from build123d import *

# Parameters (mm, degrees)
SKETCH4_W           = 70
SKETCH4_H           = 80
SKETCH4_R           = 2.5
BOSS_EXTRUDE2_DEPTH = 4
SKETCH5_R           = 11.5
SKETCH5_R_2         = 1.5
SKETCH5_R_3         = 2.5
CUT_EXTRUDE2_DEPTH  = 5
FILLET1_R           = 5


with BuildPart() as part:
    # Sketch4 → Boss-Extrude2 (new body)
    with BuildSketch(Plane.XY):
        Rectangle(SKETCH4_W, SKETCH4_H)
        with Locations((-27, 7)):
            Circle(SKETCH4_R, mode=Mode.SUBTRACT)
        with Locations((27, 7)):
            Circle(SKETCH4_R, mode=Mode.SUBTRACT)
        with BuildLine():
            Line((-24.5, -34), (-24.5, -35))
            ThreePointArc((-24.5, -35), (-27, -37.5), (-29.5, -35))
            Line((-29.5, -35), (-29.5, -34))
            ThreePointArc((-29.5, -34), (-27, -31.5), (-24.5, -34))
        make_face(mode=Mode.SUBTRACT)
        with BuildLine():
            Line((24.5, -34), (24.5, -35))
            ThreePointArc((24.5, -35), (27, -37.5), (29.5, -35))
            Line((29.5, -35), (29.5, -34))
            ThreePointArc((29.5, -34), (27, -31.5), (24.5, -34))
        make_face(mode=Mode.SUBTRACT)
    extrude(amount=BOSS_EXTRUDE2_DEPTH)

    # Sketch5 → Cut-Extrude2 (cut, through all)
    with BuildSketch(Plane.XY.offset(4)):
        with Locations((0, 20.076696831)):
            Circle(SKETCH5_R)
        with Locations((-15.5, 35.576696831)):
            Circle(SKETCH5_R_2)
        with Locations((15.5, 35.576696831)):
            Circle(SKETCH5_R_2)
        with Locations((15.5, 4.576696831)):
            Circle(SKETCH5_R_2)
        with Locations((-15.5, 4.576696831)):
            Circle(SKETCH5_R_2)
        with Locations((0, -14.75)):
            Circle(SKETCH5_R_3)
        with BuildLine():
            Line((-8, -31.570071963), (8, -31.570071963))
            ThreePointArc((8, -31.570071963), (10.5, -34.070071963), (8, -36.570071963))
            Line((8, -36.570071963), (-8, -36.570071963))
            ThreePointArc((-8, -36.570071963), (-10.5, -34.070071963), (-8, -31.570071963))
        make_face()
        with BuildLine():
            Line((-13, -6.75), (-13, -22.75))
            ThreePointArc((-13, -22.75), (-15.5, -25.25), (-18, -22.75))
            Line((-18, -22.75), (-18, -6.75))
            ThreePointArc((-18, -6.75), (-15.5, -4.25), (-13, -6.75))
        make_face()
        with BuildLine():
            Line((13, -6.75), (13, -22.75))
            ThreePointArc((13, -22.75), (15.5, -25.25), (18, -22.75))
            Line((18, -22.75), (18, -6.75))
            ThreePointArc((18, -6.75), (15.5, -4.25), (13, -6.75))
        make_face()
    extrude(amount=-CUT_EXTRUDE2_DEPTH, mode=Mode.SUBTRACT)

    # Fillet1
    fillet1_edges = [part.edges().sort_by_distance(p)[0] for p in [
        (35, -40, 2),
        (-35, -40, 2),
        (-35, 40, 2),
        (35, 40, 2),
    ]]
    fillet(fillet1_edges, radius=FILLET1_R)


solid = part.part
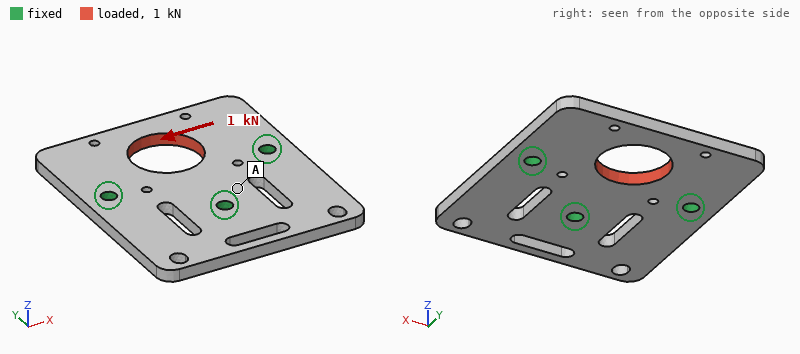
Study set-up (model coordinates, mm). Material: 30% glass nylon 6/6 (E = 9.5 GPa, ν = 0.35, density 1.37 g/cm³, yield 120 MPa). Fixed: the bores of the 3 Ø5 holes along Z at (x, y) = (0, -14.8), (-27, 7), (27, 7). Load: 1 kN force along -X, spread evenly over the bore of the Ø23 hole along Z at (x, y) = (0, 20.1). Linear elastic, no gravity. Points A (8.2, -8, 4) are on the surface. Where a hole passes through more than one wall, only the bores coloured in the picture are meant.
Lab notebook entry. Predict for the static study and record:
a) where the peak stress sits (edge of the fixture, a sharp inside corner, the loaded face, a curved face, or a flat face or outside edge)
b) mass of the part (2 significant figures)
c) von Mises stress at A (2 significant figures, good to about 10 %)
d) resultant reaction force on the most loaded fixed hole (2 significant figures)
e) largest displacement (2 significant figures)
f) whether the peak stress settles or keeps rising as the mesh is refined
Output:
edge of the fixture
26 g
1.9 MPa
510 N
52 µm
keeps rising
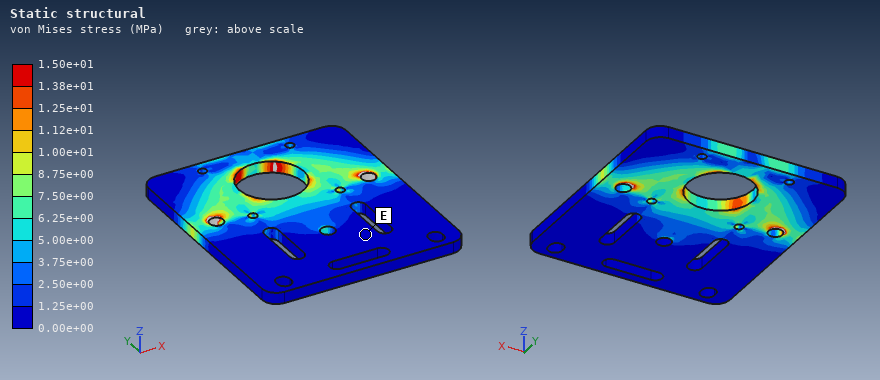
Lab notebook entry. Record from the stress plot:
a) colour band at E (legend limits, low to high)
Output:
0.00e+00 to 1.25e+00 MPa
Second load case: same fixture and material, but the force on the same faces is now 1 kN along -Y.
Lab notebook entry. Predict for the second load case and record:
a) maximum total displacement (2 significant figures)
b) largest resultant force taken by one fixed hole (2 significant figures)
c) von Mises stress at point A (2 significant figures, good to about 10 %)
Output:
33 µm
360 N
2.8 MPa
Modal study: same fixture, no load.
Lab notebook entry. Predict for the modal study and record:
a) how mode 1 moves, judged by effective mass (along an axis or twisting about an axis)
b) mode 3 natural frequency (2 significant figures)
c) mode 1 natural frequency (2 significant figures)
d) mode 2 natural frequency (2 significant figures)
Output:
along Z
1600 Hz
1400 Hz
1600 Hz
